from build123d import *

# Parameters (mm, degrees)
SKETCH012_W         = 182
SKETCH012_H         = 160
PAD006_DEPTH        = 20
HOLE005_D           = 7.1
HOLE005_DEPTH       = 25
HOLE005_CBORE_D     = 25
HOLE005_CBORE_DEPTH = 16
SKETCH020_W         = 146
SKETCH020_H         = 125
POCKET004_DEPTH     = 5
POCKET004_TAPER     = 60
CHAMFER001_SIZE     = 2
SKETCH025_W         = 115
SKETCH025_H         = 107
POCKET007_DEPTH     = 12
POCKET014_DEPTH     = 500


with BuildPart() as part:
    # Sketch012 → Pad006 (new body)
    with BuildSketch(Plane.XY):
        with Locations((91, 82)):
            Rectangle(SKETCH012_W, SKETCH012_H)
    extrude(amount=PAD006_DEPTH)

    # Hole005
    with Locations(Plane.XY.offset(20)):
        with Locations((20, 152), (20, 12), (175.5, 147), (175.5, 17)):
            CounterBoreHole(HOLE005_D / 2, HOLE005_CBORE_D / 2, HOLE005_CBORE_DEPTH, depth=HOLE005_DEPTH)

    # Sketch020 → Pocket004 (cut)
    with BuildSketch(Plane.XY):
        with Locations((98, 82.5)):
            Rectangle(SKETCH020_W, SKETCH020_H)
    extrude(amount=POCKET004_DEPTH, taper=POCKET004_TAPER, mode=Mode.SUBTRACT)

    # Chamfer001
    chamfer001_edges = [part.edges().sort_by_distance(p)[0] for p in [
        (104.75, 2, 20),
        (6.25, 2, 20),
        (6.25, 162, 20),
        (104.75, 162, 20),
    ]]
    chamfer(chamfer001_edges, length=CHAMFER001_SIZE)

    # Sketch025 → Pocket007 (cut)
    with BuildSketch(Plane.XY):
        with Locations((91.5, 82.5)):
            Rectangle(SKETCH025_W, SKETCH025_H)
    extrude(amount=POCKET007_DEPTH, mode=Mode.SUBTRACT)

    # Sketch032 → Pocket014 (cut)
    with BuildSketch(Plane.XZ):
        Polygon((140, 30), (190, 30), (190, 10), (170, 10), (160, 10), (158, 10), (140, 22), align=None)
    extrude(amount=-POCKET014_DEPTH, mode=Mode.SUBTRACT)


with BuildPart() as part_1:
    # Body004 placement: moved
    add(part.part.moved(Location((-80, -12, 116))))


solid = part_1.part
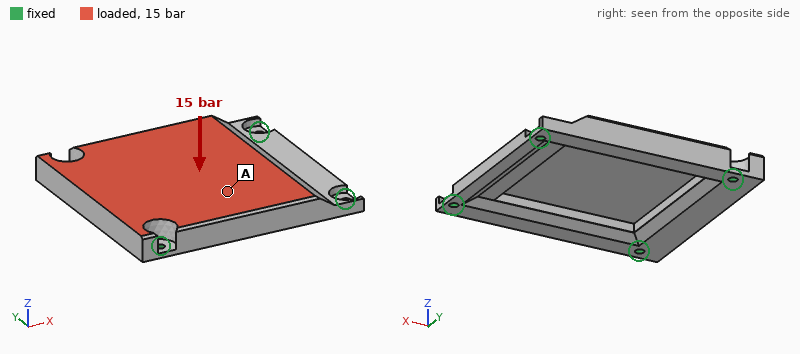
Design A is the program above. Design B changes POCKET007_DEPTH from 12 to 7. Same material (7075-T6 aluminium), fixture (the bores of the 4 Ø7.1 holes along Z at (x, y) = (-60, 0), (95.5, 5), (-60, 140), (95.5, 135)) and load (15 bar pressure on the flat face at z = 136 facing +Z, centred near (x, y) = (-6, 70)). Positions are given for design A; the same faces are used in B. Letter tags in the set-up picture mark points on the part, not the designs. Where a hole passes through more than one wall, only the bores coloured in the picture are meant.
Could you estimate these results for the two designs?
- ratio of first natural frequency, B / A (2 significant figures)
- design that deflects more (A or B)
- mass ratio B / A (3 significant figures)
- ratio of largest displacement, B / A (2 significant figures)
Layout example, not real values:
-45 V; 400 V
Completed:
0.91; A; 1.18; 0.74
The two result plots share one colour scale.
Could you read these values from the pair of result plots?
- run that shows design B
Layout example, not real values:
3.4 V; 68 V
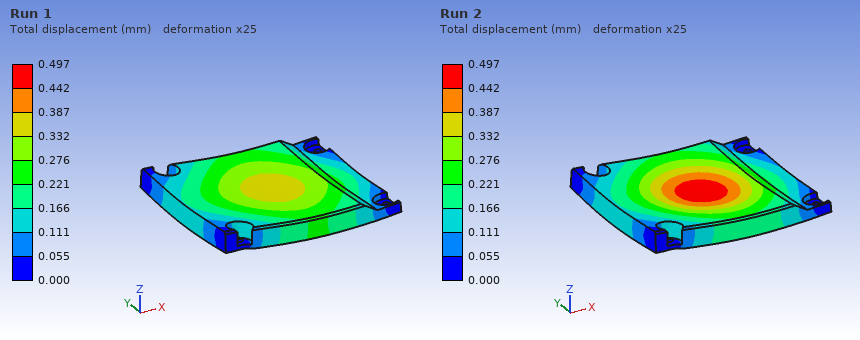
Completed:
Run 1
